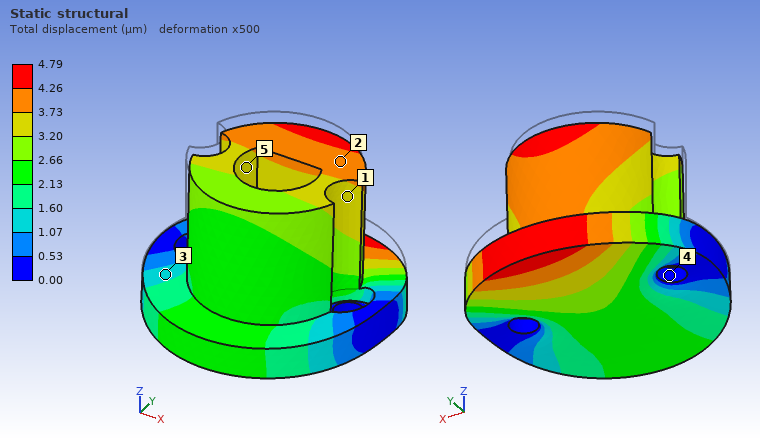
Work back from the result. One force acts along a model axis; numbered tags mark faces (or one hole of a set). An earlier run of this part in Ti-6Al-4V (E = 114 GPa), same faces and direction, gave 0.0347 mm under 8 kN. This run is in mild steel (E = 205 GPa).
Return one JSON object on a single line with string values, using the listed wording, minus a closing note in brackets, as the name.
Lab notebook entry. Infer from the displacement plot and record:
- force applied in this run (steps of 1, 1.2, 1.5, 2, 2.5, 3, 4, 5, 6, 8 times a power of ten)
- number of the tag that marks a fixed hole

{"force applied in this run": "2 kN", "number of the tag that marks a fixed hole": "4"}
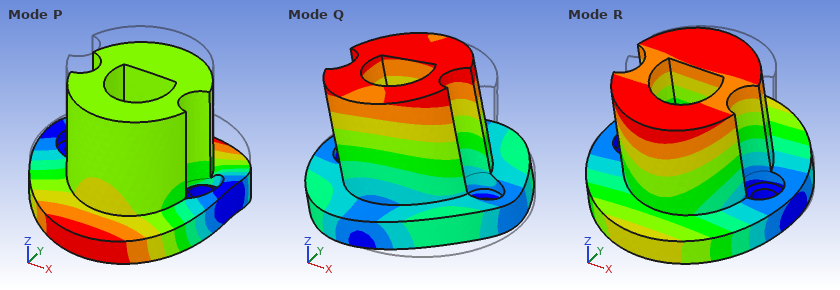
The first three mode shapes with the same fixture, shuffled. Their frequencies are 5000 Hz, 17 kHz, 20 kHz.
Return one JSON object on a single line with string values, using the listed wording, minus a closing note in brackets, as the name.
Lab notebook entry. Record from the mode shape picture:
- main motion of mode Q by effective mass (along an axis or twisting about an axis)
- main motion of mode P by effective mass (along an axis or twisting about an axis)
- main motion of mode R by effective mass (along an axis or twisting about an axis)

{"main motion of mode Q by effective mass": "along X", "main motion of mode P by effective mass": "along Z", "main motion of mode R by effective mass": "along Y"}
